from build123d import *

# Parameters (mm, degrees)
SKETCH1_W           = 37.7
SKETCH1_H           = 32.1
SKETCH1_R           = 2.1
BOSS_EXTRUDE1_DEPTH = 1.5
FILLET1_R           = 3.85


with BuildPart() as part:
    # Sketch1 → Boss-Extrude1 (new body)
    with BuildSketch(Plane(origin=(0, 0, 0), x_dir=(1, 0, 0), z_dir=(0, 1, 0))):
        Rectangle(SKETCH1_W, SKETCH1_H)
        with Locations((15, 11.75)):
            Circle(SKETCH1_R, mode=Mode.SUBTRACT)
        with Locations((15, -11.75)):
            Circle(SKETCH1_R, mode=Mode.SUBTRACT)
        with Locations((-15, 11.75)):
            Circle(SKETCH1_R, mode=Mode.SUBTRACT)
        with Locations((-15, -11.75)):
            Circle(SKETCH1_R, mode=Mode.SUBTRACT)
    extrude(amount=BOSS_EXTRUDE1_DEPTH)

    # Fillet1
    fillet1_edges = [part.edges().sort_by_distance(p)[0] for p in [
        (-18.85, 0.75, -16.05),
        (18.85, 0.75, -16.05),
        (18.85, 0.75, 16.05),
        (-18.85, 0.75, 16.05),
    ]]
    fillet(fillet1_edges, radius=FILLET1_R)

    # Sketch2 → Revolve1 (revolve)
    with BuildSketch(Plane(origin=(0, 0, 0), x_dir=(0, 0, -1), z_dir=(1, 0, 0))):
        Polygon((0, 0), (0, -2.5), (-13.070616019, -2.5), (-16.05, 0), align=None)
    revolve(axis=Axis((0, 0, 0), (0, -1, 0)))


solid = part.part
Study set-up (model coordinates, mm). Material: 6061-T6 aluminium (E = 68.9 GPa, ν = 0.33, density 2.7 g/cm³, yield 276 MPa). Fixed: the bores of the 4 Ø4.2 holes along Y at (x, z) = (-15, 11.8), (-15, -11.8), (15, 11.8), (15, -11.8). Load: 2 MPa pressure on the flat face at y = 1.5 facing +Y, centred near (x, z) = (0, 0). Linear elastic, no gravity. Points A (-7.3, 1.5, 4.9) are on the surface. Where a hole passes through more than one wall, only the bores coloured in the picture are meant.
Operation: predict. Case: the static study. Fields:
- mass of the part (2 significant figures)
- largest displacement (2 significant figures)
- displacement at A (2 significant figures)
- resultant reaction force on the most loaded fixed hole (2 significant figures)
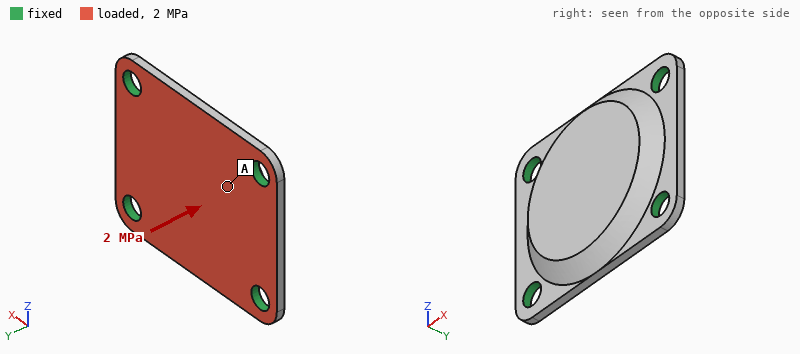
9.1 g
34 µm
26 µm
780 N
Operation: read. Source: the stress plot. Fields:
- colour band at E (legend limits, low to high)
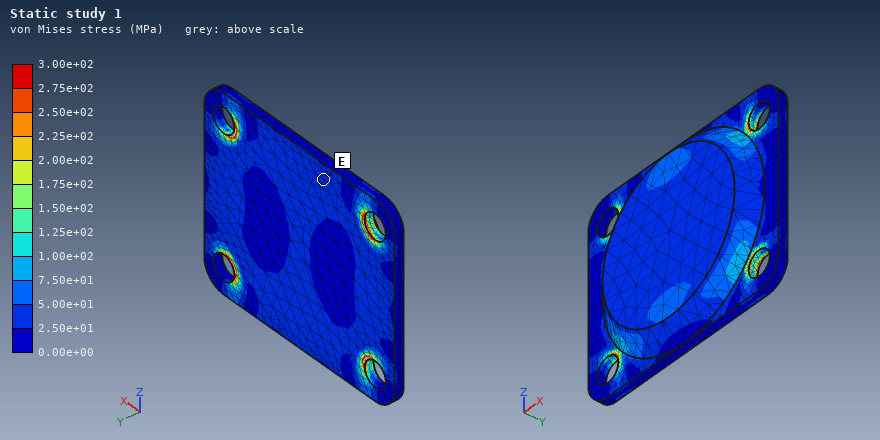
2.50e+01 to 5.00e+01 MPa
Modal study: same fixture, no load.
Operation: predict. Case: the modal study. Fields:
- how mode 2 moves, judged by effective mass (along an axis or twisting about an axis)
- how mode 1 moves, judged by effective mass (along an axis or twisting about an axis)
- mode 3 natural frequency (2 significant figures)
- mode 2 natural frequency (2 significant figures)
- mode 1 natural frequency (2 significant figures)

twisting about X
along Y
25 kHz
19 kHz
14 kHz
